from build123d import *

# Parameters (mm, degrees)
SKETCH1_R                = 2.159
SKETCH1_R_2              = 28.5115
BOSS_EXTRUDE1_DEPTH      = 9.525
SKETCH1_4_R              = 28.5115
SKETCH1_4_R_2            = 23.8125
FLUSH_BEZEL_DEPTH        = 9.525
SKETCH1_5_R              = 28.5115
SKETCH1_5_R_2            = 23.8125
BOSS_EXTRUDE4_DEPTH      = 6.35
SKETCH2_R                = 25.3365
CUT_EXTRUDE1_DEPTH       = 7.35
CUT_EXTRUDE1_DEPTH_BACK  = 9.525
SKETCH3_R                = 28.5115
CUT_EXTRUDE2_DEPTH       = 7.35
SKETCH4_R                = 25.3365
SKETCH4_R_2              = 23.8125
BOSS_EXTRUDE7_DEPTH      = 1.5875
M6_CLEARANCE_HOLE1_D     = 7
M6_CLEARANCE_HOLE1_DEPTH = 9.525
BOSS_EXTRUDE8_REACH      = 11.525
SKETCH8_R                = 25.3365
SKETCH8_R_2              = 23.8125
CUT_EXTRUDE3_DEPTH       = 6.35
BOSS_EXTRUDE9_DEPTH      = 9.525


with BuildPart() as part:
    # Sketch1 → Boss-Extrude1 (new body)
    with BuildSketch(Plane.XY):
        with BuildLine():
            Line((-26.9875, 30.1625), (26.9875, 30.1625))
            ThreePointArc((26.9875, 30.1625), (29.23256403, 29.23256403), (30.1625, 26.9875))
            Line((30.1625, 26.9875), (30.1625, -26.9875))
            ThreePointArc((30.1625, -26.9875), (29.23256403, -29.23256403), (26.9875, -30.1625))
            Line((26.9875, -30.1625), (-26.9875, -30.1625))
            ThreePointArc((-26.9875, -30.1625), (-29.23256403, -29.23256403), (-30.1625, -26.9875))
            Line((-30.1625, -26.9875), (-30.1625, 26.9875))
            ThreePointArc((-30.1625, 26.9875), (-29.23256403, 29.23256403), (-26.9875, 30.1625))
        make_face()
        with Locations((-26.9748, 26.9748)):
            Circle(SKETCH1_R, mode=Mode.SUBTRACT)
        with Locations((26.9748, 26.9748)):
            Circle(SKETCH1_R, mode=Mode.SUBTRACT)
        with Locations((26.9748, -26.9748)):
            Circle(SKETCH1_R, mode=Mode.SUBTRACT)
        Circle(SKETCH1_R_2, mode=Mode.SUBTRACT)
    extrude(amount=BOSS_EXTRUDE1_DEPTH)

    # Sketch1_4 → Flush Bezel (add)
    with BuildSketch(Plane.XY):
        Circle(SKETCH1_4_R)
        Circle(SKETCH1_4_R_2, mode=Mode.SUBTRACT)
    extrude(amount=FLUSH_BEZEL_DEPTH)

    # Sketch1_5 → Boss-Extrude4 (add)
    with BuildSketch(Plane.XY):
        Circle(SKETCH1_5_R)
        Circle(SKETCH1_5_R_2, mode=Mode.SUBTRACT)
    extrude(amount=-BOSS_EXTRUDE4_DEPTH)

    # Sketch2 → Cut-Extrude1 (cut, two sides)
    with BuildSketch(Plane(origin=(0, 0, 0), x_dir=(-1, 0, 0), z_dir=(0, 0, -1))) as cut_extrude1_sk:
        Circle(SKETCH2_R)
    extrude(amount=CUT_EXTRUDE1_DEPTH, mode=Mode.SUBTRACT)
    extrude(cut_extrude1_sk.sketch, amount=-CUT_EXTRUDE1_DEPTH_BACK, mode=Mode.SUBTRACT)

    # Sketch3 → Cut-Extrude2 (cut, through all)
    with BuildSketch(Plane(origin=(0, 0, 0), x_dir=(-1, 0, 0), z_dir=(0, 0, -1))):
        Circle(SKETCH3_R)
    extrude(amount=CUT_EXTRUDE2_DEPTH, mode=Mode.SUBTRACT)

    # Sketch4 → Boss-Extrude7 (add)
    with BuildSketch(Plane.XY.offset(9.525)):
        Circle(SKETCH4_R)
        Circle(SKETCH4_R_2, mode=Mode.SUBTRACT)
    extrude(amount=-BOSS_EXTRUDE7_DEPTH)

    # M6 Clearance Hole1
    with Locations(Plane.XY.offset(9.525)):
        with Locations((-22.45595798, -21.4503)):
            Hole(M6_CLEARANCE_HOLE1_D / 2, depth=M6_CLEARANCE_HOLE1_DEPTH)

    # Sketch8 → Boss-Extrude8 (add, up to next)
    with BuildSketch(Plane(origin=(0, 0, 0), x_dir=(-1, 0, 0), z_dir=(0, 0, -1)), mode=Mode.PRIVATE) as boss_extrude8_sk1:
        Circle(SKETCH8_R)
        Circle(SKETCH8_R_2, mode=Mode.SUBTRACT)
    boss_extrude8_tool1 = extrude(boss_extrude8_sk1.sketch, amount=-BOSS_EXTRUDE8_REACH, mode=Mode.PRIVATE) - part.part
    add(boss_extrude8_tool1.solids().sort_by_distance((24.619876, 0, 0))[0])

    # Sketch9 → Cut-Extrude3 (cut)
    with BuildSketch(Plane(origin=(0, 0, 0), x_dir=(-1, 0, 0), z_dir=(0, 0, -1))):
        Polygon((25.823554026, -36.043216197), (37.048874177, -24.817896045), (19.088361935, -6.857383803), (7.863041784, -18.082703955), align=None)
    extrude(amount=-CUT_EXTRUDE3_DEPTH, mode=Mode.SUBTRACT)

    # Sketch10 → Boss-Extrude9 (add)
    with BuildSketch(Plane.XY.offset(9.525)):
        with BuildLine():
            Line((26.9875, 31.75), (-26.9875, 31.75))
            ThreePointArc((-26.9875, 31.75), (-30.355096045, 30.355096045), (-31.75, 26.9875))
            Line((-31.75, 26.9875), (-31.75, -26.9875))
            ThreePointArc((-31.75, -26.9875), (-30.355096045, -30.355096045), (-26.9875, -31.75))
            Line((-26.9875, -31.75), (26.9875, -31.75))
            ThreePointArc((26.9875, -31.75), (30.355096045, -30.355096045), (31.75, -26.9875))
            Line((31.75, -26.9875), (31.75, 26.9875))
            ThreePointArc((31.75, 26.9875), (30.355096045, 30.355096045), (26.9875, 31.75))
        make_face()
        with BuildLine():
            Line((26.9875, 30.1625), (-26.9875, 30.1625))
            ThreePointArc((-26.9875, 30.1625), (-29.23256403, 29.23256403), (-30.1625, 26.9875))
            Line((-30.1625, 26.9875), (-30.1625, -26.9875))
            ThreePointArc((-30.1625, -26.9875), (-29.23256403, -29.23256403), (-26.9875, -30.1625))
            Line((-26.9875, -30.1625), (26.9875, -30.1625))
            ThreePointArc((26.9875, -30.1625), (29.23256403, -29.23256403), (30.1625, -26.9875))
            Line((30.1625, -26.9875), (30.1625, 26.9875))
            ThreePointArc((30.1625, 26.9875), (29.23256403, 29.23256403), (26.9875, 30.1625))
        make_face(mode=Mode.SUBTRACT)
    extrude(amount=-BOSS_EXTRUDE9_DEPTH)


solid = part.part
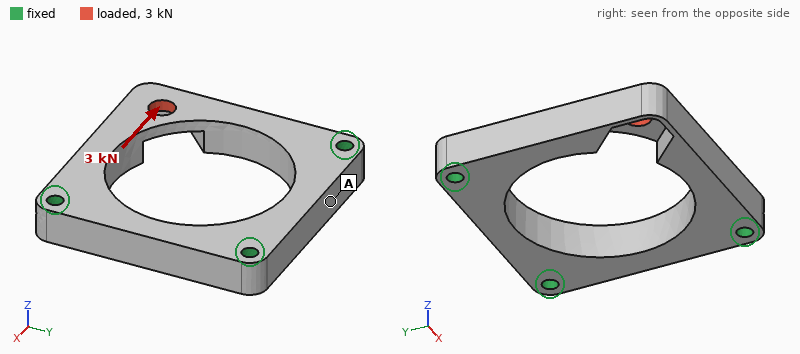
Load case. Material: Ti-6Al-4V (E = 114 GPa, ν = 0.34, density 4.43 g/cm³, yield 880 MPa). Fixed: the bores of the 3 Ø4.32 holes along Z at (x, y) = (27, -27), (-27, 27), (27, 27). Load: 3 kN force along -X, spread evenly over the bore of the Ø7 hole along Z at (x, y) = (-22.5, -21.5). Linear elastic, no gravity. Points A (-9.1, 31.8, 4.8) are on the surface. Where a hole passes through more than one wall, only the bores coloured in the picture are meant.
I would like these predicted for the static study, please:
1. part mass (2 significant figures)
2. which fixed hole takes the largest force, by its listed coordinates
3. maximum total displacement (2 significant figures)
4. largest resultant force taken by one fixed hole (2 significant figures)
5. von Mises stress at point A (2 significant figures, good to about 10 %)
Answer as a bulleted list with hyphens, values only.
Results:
- 85 g
- (27, -27)
- 80 µm
- 2.6 kN
- 13 MPa
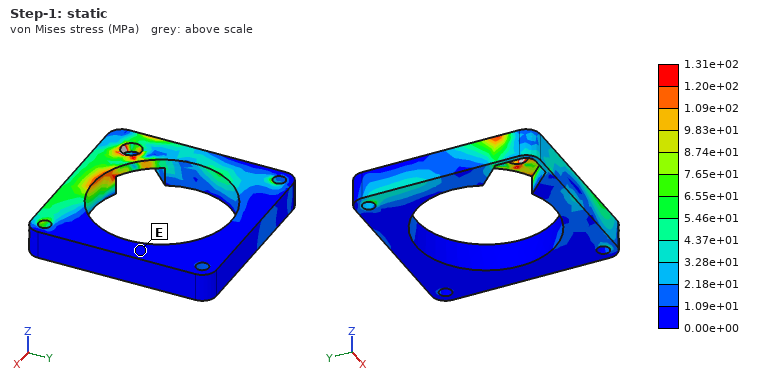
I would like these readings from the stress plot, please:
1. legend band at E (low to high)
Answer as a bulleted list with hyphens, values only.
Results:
- 0.00e+00 to 1.09e+01 MPa
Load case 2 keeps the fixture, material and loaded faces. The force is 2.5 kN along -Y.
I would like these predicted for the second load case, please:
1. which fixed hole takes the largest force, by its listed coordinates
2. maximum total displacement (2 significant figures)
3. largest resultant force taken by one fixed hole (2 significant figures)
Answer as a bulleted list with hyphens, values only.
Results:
- (-27, 27)
- 66 µm
- 2.2 kN
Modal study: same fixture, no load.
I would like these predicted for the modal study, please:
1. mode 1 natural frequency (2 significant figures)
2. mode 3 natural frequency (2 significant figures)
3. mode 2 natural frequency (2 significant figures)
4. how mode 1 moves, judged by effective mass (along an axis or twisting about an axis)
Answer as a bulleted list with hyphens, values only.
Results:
- 3800 Hz
- 10 kHz
- 9300 Hz
- along Z
